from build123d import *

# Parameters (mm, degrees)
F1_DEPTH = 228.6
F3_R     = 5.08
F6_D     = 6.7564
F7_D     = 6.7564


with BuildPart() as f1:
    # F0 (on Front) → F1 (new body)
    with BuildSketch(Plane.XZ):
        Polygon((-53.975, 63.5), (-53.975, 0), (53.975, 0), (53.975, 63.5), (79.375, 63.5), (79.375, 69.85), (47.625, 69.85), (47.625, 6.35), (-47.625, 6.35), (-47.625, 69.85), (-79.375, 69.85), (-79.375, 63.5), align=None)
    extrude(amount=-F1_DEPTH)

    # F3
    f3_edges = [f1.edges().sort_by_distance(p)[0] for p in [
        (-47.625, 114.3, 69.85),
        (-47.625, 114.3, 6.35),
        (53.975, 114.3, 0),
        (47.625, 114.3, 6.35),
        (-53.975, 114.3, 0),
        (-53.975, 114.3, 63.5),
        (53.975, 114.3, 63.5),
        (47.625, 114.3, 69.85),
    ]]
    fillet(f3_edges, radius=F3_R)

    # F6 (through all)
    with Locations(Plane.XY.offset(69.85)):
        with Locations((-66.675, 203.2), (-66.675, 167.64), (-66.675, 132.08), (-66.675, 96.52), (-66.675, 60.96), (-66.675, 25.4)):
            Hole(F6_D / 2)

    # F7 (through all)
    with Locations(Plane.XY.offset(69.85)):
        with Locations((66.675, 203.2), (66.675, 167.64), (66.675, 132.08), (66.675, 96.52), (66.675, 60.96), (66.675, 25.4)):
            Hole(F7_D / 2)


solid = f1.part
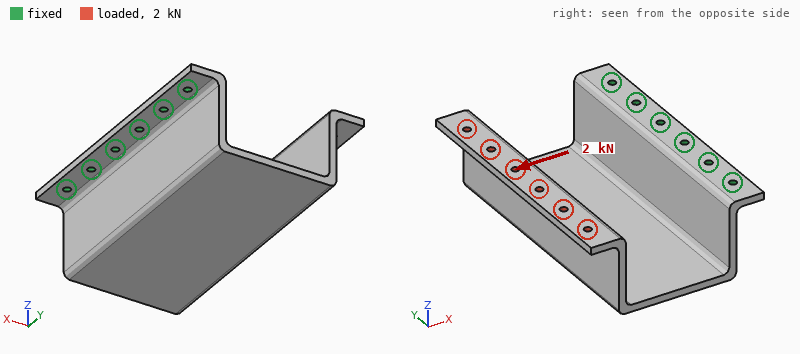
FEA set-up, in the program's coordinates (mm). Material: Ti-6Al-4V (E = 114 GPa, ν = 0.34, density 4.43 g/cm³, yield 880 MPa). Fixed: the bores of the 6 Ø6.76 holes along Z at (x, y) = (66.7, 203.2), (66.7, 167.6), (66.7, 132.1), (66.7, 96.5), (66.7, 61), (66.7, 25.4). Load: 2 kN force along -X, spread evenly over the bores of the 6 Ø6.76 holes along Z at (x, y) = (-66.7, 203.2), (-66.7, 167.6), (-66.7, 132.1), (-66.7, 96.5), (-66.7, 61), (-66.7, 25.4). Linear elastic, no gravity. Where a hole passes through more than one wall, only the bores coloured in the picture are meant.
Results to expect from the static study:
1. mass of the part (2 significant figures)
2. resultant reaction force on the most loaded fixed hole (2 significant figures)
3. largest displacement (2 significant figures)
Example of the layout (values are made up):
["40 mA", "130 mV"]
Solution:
["1.8 kg", "440 N", "3.1 mm"]
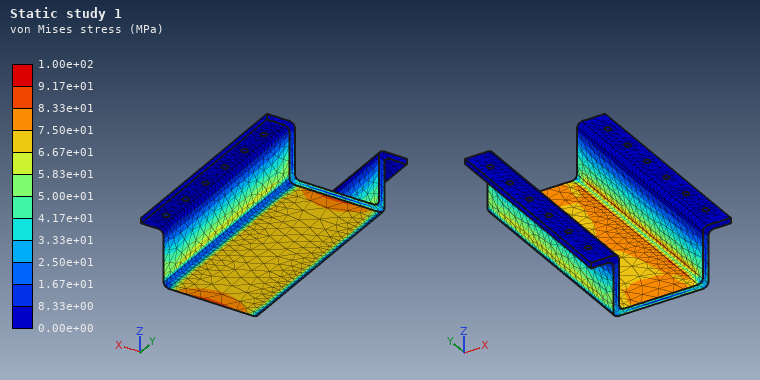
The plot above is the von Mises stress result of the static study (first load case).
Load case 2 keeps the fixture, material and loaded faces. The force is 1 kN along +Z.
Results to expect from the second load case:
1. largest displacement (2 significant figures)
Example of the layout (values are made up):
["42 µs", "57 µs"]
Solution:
["3.0 mm"]
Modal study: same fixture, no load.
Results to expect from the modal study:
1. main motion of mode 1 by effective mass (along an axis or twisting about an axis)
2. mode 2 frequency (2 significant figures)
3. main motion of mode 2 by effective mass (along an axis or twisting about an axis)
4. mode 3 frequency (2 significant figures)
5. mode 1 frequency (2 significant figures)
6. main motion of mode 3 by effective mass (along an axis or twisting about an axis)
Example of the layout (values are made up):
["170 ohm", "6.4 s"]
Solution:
["along Z", "220 Hz", "along Y", "330 Hz", "120 Hz", "along X"]
